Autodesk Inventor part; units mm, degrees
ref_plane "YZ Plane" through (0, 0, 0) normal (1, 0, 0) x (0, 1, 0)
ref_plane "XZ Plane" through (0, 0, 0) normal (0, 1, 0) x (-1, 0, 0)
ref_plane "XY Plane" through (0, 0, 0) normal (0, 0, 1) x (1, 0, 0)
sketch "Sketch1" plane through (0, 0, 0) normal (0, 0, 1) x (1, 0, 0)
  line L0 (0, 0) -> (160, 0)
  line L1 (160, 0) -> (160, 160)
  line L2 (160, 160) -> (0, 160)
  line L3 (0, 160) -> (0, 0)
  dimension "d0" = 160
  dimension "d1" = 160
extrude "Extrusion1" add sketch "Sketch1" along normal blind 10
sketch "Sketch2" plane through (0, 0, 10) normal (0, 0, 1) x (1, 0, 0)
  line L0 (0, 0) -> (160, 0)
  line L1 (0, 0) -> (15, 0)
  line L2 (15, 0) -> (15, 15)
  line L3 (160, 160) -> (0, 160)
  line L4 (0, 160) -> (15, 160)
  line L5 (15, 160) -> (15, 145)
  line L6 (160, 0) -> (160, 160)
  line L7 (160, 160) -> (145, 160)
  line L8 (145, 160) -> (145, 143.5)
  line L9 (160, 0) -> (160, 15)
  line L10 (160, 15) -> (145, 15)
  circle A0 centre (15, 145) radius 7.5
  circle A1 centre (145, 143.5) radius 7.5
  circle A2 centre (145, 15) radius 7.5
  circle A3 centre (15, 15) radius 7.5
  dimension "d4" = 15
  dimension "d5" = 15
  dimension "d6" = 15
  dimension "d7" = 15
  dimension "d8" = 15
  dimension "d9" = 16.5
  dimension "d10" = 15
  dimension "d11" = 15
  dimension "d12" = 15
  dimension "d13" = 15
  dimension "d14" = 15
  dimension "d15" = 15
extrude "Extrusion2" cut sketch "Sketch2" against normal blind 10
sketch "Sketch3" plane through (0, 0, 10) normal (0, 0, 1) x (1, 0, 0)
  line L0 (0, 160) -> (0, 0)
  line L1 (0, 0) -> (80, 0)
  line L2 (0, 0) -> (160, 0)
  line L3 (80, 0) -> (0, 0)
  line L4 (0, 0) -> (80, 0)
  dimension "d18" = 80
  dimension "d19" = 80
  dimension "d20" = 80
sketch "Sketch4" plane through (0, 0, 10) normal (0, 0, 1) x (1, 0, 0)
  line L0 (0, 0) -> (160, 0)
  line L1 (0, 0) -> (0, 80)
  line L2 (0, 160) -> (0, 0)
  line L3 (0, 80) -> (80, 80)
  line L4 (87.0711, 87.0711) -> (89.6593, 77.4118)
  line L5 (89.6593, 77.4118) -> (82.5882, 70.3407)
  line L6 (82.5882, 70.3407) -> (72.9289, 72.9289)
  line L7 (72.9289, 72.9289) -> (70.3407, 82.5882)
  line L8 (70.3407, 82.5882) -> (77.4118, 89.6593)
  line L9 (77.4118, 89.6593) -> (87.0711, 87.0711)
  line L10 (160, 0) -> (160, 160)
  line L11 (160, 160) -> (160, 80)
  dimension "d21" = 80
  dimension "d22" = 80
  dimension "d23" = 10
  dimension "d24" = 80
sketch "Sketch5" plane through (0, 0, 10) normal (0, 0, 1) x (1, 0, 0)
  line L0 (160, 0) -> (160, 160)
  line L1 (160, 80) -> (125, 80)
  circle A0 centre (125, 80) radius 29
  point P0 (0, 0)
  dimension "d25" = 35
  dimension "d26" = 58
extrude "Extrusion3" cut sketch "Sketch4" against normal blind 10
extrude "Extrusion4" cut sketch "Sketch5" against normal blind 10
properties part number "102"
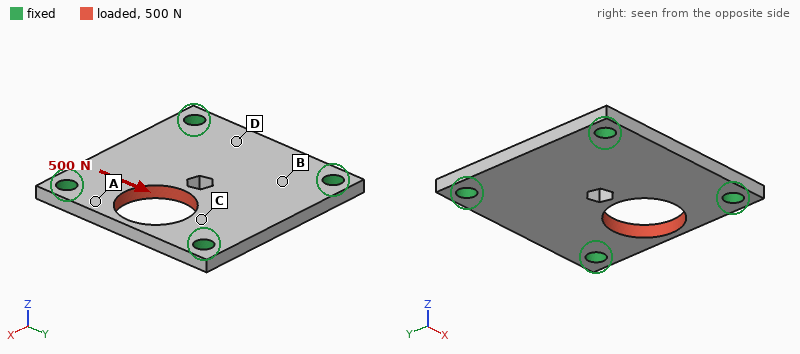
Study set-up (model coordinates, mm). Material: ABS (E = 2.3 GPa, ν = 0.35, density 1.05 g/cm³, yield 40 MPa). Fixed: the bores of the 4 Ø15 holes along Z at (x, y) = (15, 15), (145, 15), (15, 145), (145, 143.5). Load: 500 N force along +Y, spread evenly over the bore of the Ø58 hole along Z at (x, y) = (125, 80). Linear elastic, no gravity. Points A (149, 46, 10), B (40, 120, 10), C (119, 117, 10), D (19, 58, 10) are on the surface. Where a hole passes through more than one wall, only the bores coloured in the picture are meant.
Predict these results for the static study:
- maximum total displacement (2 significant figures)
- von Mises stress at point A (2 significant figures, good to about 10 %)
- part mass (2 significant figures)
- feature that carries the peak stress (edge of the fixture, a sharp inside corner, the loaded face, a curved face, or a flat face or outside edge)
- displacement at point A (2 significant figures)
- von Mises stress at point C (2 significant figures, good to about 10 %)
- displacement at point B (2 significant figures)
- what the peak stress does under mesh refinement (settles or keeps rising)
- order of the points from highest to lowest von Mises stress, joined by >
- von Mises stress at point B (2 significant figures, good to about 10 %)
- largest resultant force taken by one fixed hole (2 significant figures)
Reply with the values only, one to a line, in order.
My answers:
13 µm
0.44 MPa
230 g
edge of the fixture
5.5 µm
0.34 MPa
3.2 µm
keeps rising
A > C > B > D
0.18 MPa
190 N
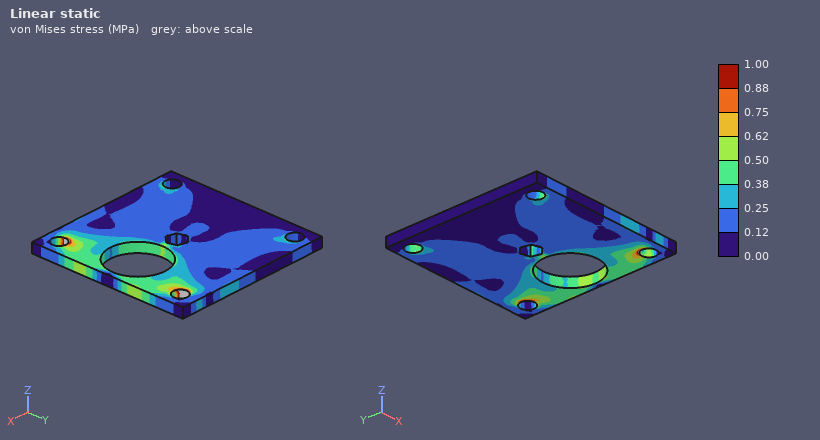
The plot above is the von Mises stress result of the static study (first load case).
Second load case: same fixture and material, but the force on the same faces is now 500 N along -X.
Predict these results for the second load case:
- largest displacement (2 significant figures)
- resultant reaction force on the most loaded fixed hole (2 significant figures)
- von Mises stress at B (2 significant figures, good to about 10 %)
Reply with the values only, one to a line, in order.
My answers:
63 µm
150 N
0.23 MPa
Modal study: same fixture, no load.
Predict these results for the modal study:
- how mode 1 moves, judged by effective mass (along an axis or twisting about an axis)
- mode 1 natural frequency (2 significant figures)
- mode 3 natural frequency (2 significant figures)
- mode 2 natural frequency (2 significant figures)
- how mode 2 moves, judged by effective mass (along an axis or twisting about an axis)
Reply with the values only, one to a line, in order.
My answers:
along Z
670 Hz
1100 Hz
1100 Hz
twisting about X
